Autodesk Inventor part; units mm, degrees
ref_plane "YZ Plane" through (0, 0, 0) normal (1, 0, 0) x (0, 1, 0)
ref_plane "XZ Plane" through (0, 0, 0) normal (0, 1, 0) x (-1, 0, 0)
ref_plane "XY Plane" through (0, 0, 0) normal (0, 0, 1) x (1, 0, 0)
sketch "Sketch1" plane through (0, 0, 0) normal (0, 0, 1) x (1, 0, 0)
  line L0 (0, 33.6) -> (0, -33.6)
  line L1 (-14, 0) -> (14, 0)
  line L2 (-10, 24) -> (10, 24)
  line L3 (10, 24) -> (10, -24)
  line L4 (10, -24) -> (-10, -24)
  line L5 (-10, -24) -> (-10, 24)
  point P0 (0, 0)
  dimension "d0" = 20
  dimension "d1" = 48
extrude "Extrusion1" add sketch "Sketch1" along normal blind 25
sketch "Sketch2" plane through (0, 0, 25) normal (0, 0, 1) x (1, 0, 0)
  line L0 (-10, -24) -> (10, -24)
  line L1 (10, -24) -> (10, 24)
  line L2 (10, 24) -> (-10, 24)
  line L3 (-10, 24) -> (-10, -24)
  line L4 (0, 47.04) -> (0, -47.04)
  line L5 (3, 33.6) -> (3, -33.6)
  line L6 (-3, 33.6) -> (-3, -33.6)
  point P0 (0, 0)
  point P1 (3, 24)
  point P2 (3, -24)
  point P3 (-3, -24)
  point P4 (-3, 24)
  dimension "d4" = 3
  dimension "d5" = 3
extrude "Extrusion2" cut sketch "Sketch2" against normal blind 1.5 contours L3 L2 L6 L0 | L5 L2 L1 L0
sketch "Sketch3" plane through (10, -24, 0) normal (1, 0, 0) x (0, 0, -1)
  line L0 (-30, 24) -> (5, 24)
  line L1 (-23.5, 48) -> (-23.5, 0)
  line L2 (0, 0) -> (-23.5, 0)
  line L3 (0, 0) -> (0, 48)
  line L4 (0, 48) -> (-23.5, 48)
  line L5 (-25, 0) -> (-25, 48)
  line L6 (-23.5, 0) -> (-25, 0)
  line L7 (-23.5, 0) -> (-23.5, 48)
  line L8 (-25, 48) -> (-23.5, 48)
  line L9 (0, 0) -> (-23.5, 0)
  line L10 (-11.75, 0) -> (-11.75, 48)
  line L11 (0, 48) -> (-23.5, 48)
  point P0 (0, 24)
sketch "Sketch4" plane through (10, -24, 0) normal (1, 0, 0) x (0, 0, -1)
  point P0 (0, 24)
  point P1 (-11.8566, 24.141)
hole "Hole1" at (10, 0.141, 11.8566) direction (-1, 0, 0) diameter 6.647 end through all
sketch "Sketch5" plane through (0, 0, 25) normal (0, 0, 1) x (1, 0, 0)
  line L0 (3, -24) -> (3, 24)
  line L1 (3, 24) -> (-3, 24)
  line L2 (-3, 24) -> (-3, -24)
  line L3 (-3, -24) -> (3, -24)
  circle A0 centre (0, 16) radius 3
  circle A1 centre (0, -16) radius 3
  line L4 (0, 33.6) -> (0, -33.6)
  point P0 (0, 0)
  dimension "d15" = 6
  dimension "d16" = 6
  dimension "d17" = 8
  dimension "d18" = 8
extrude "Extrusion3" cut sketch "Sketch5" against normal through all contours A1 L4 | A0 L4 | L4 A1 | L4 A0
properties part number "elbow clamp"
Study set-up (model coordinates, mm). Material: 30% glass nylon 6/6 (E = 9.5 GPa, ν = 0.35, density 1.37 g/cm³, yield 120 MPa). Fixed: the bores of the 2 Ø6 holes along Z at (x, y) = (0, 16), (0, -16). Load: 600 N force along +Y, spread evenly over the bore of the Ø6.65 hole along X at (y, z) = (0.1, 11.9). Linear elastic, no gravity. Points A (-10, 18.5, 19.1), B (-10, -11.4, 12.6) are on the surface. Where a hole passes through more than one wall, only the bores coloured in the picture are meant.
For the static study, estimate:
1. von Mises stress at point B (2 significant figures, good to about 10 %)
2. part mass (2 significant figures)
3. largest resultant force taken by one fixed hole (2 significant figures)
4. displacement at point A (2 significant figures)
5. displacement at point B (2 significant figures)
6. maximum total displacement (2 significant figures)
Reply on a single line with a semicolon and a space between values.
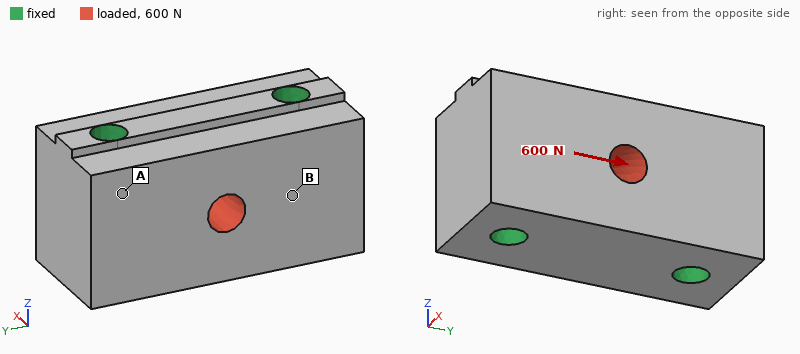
0.61 MPa; 29 g; 300 N; 0.46 µm; 0.79 µm; 1.7 µm
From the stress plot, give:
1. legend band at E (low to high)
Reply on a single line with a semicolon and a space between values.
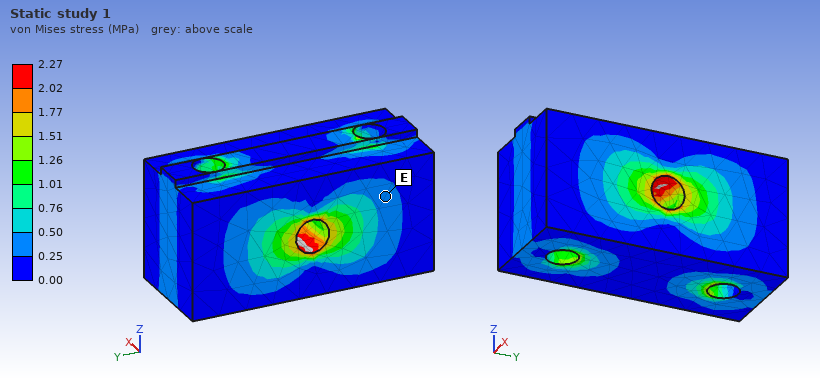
0.25 to 0.50 MPa
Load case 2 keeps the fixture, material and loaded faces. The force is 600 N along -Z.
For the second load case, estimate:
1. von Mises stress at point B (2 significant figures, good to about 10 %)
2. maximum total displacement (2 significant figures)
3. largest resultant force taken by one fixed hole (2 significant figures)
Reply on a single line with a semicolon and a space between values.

0.87 MPa; 3.7 µm; 300 N
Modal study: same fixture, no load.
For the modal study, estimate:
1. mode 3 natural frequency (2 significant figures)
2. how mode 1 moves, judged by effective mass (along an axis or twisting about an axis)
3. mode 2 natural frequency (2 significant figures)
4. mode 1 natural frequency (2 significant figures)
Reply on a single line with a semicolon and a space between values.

24 kHz; along X; 23 kHz; 20 kHz
